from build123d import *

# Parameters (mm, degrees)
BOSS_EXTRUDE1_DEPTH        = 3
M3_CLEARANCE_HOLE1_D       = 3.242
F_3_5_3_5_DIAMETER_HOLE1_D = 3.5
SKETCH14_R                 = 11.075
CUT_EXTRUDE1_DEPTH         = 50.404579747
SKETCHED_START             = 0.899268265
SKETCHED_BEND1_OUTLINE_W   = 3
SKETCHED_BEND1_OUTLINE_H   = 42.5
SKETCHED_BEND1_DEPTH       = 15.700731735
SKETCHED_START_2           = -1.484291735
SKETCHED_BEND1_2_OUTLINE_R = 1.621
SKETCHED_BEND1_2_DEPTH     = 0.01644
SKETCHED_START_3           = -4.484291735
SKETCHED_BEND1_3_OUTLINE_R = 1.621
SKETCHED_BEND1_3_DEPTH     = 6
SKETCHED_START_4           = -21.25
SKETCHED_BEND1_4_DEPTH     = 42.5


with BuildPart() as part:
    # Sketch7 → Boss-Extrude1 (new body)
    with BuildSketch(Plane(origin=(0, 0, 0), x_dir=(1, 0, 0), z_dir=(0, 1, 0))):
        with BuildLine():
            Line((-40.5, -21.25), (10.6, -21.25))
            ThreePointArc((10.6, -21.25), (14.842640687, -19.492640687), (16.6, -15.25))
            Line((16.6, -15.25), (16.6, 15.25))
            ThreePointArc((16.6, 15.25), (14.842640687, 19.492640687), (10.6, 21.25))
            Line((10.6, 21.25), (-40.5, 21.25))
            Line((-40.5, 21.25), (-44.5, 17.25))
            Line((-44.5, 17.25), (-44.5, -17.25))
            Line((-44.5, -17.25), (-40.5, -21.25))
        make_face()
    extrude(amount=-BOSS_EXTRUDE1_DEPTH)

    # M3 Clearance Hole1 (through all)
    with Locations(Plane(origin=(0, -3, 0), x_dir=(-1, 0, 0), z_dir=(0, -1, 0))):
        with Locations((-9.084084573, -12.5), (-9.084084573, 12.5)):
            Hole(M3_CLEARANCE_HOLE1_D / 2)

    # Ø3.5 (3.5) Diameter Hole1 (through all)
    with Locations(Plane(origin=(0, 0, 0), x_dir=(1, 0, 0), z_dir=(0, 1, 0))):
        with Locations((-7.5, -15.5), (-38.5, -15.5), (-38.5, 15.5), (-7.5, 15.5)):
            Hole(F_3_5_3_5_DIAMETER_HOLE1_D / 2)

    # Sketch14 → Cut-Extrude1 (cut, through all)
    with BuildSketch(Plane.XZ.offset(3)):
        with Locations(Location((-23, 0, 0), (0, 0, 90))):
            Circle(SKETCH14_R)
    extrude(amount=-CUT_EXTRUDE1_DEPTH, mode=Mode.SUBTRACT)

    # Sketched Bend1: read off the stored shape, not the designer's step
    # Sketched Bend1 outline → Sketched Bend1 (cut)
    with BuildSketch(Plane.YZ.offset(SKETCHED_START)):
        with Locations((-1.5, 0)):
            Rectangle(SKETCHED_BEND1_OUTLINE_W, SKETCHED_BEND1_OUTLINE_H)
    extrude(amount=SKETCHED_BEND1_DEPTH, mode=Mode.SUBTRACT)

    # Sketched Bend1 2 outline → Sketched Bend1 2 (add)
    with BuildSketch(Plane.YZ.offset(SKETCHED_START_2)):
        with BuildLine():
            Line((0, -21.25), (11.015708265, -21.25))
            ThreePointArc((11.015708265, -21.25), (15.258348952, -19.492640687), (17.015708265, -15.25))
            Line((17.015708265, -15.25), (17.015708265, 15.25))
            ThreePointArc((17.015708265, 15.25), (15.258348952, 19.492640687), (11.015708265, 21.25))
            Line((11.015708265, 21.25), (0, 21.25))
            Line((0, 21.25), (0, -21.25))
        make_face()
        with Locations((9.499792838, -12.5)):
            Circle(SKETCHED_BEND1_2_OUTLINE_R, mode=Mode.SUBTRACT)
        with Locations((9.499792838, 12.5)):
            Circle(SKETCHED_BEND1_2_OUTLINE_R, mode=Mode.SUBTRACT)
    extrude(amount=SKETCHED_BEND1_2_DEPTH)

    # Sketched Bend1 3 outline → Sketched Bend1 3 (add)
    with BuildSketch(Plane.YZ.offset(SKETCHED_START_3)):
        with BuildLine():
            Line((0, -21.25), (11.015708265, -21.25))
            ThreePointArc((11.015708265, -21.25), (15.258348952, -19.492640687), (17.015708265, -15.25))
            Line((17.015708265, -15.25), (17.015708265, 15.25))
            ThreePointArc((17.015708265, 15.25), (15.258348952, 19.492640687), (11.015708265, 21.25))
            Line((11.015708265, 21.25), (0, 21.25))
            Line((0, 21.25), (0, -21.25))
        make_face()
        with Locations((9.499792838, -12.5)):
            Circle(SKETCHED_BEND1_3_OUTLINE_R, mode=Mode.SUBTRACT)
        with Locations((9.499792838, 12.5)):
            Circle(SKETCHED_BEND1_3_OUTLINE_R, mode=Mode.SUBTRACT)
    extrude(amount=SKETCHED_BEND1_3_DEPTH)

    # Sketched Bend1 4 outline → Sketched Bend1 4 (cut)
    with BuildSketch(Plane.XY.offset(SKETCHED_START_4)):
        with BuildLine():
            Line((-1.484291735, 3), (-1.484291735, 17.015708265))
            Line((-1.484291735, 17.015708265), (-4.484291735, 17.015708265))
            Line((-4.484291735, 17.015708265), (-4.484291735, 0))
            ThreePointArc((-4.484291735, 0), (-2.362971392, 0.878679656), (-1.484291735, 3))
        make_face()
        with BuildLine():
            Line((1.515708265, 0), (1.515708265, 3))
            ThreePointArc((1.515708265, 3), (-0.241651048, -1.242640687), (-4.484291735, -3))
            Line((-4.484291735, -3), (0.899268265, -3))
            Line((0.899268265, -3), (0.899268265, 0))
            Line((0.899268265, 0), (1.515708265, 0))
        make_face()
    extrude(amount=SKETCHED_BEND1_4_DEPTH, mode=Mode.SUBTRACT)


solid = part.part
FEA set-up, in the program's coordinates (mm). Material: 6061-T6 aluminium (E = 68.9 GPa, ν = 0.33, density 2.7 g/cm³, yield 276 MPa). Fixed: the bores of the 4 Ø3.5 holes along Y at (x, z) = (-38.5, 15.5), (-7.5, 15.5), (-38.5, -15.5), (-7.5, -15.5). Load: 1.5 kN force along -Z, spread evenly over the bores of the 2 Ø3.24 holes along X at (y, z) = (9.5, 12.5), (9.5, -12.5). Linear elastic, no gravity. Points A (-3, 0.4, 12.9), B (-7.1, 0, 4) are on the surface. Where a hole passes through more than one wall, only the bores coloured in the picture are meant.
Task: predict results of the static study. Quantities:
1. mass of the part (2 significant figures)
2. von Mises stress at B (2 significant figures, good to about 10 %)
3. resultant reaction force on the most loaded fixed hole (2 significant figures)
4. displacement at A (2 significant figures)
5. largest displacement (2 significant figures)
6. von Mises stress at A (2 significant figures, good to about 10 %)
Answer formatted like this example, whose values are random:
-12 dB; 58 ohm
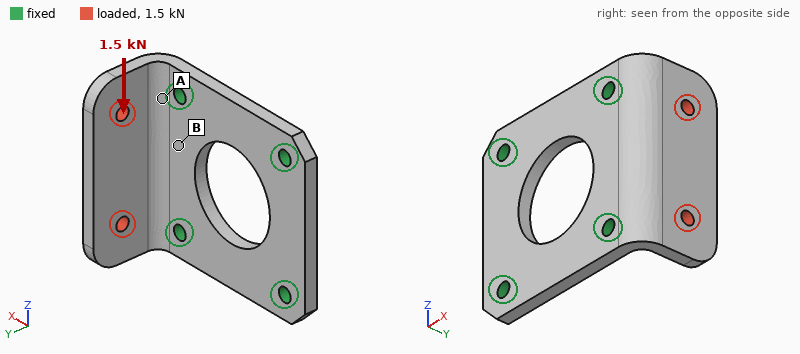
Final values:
17 g; 26 MPa; 950 N; 9.6 µm; 56 µm; 73 MPa
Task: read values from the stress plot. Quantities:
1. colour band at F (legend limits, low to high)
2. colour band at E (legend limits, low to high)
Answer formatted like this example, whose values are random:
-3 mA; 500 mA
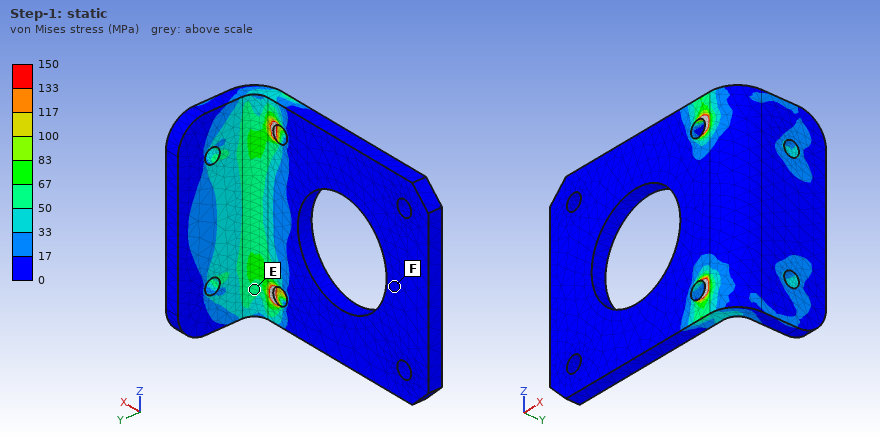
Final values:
0 to 17 MPa; 50 to 67 MPa
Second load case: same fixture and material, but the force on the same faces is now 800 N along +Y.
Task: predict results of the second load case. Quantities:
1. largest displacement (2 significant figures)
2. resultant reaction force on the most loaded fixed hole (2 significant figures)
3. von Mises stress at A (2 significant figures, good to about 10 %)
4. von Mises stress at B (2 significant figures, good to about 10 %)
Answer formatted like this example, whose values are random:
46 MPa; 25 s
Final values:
81 µm; 410 N; 37 MPa; 20 MPa
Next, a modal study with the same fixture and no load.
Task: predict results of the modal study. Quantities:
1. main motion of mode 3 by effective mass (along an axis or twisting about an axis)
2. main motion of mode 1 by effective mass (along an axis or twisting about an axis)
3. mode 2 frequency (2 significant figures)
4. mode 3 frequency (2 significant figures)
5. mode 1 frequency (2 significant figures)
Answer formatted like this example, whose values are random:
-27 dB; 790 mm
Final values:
along Y; along X; 8100 Hz; 15 kHz; 4700 Hz
